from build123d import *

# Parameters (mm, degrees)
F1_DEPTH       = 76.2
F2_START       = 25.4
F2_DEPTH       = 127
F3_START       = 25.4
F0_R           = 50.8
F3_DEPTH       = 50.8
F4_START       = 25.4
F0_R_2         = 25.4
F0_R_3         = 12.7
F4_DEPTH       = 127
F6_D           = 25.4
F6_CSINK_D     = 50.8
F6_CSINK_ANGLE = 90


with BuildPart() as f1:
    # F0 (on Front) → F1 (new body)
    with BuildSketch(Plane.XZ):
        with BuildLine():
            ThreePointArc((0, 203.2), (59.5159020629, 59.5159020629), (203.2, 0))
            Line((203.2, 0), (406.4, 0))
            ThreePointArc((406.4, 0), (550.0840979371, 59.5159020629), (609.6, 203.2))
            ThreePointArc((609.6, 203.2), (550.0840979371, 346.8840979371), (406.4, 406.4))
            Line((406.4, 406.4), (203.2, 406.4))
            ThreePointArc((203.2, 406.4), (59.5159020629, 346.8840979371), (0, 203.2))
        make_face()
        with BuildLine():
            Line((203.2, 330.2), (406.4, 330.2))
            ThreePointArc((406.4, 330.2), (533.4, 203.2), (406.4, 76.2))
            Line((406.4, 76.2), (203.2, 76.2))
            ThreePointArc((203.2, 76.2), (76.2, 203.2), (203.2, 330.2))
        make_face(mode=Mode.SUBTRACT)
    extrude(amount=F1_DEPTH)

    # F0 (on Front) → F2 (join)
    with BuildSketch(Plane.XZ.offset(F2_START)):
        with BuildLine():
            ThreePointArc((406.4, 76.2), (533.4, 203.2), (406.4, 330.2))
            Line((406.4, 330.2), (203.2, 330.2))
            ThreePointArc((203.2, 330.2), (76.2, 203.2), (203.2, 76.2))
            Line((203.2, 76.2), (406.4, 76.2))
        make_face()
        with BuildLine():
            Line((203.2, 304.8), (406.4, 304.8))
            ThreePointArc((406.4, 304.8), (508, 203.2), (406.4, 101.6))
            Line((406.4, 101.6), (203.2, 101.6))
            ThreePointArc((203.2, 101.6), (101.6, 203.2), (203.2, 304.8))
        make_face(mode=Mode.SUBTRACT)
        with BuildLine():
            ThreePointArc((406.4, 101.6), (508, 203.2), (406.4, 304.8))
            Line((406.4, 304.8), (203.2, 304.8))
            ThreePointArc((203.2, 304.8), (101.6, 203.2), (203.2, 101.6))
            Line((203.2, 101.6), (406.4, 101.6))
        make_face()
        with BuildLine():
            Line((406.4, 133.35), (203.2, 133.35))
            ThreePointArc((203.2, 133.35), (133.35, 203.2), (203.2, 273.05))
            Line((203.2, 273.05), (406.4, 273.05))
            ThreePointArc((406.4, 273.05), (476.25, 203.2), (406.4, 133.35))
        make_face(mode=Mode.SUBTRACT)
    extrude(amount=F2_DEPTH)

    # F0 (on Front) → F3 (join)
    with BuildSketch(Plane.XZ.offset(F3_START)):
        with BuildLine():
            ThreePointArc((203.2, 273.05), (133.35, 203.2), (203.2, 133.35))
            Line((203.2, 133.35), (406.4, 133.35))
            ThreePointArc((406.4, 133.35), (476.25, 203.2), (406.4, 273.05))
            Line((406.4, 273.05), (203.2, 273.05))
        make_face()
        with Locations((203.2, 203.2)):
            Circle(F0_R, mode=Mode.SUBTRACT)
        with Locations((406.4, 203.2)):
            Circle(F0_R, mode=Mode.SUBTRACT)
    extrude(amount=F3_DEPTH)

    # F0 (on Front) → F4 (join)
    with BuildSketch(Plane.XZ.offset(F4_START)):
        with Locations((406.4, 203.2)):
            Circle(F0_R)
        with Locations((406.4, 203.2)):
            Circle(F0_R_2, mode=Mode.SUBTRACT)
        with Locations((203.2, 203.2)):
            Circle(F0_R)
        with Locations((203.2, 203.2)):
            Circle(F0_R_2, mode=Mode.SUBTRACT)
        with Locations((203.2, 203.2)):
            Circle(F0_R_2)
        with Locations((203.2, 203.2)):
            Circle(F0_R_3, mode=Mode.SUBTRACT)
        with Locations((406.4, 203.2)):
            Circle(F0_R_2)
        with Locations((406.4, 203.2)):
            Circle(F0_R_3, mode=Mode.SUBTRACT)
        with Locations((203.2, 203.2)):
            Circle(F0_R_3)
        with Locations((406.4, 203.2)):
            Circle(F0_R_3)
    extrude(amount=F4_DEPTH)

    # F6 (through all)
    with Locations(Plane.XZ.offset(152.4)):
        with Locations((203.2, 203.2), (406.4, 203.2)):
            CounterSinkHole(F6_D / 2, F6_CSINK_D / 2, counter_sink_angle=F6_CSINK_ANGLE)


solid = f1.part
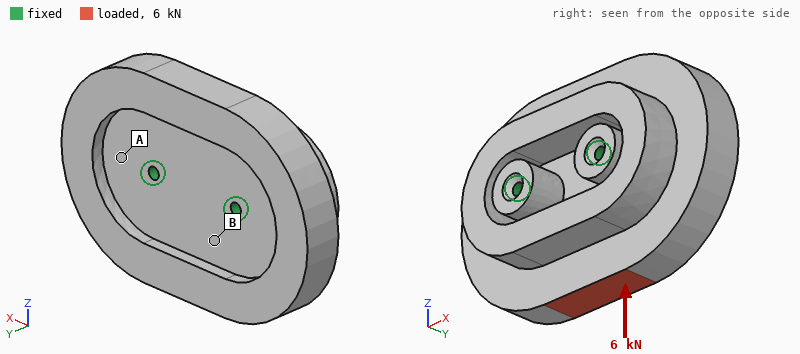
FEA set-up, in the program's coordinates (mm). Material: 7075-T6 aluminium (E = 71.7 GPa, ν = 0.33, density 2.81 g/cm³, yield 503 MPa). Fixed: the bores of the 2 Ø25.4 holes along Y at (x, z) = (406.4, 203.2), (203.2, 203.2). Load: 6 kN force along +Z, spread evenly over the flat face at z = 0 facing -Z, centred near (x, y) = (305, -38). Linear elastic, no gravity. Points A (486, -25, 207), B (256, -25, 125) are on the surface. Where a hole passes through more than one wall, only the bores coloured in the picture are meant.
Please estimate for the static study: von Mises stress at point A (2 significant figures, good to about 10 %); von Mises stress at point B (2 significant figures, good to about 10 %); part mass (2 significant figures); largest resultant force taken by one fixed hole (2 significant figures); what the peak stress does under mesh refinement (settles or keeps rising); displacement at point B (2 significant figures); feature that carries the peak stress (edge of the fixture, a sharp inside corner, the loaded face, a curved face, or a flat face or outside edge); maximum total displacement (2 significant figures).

0.14 MPa
0.67 MPa
54 kg
3.1 kN
keeps rising
1.3 µm
edge of the fixture
4.5 µm
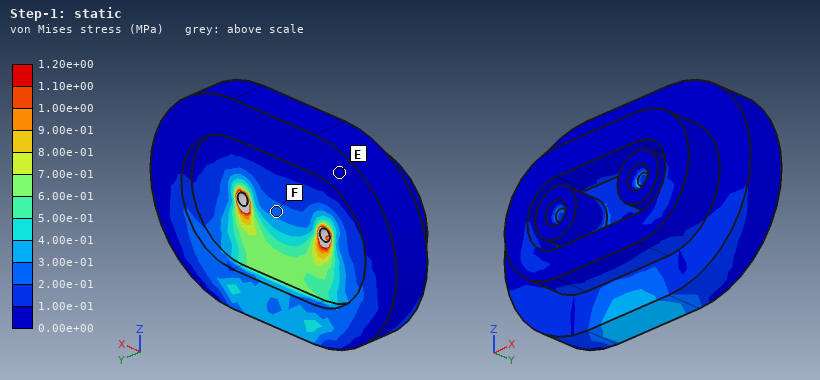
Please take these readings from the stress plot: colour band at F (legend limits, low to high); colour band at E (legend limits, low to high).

2.00e-01 to 3.00e-01 MPa
0.00e+00 to 1.00e-01 MPa
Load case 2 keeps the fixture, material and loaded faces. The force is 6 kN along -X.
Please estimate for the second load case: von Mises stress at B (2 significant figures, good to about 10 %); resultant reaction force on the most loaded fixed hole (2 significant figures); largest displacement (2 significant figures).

0.72 MPa
6.2 kN
3.9 µm
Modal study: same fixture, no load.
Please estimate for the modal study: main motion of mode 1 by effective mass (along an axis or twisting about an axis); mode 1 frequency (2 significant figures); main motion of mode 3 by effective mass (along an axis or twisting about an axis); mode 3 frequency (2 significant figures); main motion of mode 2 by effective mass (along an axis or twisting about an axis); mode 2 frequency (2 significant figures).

twisting about X
780 Hz
twisting about Y
1300 Hz
twisting about Z
1200 Hz
